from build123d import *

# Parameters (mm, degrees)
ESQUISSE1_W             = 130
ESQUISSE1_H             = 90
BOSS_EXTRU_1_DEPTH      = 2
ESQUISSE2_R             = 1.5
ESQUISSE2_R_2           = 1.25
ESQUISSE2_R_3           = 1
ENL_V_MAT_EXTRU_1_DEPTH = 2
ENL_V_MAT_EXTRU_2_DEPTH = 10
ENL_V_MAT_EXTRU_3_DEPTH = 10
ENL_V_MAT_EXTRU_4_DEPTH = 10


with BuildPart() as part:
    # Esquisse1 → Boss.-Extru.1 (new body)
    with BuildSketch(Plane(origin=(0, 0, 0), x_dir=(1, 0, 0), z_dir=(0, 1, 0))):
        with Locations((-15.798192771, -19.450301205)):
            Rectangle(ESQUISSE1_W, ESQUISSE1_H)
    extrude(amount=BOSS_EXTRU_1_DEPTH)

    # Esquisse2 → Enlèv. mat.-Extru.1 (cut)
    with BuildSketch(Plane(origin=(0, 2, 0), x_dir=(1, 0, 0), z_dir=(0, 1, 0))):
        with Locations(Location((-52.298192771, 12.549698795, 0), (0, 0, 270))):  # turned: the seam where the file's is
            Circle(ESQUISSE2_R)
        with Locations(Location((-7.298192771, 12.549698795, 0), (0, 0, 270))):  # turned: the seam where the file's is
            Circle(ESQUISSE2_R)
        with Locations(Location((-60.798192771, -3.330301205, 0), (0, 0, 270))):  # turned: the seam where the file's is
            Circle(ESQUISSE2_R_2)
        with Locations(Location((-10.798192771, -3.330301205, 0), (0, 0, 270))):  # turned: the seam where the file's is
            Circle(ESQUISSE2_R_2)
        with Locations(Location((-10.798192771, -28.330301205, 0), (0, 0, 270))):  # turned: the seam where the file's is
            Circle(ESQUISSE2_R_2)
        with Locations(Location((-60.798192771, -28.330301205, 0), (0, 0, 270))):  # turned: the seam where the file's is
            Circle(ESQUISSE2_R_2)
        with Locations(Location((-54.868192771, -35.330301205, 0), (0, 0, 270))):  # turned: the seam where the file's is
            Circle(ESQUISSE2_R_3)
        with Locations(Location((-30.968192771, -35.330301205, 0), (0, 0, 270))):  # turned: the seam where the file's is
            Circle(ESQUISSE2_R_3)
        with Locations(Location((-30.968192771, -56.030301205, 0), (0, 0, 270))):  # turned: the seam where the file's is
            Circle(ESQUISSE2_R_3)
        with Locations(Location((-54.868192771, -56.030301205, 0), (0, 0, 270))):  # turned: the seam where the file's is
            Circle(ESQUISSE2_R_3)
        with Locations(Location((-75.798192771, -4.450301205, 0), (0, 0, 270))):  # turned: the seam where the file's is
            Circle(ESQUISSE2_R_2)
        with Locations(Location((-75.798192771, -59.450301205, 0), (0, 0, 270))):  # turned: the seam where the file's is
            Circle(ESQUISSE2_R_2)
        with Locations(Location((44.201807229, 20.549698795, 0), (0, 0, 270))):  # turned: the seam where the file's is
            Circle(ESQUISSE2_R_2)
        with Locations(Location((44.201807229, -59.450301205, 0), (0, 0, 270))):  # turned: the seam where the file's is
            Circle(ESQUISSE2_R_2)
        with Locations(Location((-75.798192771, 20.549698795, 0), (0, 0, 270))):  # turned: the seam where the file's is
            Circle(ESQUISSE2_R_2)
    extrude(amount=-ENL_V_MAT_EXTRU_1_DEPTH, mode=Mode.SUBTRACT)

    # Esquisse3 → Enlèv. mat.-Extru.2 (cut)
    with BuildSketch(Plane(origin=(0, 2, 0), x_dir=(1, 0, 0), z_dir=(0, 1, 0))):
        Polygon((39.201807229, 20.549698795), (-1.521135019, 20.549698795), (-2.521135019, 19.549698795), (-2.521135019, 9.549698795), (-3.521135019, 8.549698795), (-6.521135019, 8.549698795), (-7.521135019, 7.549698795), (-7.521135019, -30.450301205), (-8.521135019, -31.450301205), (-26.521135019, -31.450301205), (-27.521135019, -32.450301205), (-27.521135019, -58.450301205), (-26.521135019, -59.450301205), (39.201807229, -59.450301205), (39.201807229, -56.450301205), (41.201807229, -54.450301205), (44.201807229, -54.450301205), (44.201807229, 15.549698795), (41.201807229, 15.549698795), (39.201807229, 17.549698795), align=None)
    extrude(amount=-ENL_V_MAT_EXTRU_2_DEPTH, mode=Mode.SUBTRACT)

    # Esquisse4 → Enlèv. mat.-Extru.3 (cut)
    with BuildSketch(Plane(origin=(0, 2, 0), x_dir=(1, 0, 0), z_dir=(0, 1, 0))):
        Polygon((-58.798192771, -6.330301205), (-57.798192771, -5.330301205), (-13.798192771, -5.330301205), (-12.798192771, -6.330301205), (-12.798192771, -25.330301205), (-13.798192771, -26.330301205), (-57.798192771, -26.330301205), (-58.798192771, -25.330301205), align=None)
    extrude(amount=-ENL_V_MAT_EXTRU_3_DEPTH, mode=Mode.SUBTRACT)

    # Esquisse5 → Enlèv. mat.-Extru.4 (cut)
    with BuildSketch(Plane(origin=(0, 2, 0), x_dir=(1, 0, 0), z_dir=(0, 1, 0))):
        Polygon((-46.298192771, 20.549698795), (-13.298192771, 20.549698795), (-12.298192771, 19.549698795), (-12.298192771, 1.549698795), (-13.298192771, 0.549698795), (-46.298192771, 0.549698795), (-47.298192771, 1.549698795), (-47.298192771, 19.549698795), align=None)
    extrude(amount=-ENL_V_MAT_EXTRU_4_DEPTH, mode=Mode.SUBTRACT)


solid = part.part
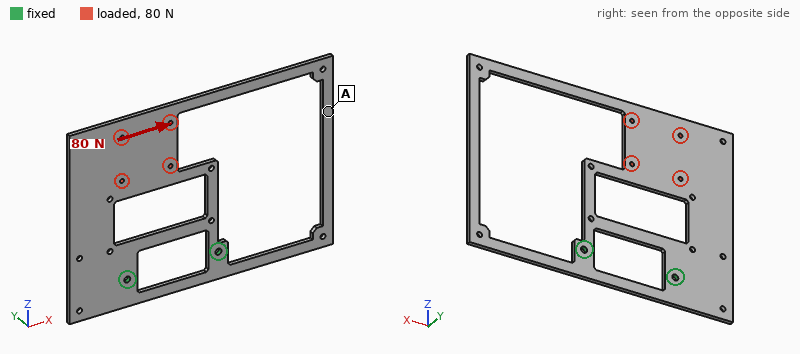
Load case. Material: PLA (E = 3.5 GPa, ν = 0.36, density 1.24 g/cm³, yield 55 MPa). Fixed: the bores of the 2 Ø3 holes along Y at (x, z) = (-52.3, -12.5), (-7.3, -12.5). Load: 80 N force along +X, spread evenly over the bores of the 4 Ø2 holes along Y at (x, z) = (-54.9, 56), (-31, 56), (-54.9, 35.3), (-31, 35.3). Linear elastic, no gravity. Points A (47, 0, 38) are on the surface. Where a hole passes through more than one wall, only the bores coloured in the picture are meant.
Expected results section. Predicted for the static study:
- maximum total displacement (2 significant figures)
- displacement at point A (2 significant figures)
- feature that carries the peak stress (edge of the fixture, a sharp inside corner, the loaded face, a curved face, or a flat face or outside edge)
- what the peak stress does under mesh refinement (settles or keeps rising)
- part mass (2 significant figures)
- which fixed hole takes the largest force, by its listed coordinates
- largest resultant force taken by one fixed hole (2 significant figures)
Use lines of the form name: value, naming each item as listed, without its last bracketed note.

maximum total displacement: 1.6 mm
displacement at point A: 1.3 mm
feature that carries the peak stress: edge of the fixture
what the peak stress does under mesh refinement: keeps rising
part mass: 13 g
which fixed hole takes the largest force, by its listed coordinates: (-52.3, -12.5)
largest resultant force taken by one fixed hole: 110 N
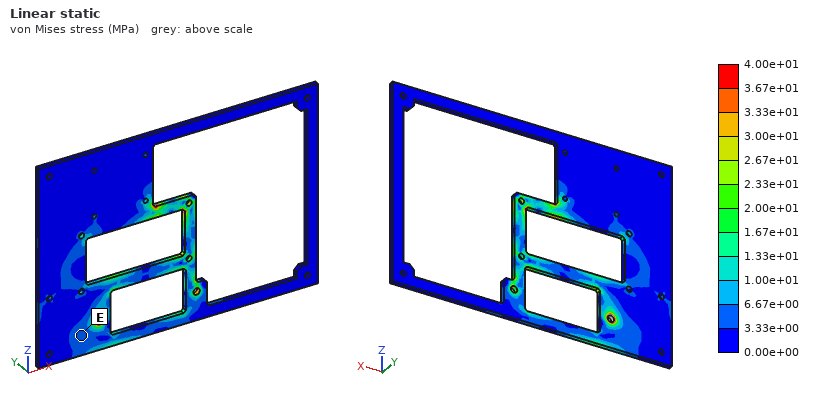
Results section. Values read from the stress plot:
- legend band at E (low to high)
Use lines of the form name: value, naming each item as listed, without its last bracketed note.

legend band at E: 3.33e+00 to 6.67e+00 MPa
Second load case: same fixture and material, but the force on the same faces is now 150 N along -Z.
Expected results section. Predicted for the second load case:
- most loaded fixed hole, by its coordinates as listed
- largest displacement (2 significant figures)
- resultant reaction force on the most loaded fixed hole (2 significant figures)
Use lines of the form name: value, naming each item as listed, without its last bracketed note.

most loaded fixed hole, by its coordinates as listed: (-52.3, -12.5)
largest displacement: 0.65 mm
resultant reaction force on the most loaded fixed hole: 110 N
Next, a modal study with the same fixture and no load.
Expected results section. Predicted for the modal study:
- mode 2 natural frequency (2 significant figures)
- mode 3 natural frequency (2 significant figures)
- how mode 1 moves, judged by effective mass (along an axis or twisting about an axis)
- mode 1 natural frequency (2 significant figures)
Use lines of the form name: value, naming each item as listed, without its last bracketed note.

mode 2 natural frequency: 71 Hz
mode 3 natural frequency: 140 Hz
how mode 1 moves, judged by effective mass: along Y
mode 1 natural frequency: 47 Hz
